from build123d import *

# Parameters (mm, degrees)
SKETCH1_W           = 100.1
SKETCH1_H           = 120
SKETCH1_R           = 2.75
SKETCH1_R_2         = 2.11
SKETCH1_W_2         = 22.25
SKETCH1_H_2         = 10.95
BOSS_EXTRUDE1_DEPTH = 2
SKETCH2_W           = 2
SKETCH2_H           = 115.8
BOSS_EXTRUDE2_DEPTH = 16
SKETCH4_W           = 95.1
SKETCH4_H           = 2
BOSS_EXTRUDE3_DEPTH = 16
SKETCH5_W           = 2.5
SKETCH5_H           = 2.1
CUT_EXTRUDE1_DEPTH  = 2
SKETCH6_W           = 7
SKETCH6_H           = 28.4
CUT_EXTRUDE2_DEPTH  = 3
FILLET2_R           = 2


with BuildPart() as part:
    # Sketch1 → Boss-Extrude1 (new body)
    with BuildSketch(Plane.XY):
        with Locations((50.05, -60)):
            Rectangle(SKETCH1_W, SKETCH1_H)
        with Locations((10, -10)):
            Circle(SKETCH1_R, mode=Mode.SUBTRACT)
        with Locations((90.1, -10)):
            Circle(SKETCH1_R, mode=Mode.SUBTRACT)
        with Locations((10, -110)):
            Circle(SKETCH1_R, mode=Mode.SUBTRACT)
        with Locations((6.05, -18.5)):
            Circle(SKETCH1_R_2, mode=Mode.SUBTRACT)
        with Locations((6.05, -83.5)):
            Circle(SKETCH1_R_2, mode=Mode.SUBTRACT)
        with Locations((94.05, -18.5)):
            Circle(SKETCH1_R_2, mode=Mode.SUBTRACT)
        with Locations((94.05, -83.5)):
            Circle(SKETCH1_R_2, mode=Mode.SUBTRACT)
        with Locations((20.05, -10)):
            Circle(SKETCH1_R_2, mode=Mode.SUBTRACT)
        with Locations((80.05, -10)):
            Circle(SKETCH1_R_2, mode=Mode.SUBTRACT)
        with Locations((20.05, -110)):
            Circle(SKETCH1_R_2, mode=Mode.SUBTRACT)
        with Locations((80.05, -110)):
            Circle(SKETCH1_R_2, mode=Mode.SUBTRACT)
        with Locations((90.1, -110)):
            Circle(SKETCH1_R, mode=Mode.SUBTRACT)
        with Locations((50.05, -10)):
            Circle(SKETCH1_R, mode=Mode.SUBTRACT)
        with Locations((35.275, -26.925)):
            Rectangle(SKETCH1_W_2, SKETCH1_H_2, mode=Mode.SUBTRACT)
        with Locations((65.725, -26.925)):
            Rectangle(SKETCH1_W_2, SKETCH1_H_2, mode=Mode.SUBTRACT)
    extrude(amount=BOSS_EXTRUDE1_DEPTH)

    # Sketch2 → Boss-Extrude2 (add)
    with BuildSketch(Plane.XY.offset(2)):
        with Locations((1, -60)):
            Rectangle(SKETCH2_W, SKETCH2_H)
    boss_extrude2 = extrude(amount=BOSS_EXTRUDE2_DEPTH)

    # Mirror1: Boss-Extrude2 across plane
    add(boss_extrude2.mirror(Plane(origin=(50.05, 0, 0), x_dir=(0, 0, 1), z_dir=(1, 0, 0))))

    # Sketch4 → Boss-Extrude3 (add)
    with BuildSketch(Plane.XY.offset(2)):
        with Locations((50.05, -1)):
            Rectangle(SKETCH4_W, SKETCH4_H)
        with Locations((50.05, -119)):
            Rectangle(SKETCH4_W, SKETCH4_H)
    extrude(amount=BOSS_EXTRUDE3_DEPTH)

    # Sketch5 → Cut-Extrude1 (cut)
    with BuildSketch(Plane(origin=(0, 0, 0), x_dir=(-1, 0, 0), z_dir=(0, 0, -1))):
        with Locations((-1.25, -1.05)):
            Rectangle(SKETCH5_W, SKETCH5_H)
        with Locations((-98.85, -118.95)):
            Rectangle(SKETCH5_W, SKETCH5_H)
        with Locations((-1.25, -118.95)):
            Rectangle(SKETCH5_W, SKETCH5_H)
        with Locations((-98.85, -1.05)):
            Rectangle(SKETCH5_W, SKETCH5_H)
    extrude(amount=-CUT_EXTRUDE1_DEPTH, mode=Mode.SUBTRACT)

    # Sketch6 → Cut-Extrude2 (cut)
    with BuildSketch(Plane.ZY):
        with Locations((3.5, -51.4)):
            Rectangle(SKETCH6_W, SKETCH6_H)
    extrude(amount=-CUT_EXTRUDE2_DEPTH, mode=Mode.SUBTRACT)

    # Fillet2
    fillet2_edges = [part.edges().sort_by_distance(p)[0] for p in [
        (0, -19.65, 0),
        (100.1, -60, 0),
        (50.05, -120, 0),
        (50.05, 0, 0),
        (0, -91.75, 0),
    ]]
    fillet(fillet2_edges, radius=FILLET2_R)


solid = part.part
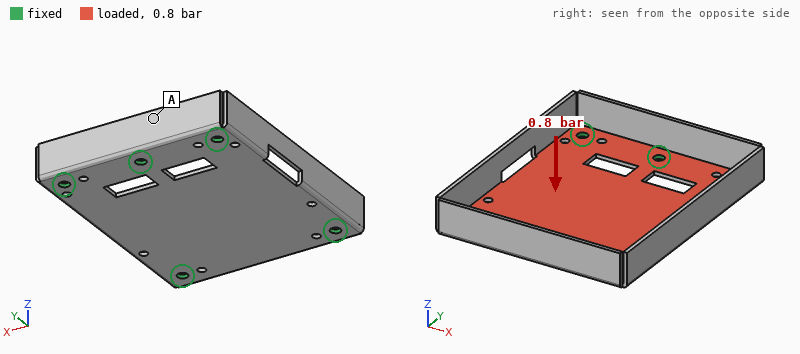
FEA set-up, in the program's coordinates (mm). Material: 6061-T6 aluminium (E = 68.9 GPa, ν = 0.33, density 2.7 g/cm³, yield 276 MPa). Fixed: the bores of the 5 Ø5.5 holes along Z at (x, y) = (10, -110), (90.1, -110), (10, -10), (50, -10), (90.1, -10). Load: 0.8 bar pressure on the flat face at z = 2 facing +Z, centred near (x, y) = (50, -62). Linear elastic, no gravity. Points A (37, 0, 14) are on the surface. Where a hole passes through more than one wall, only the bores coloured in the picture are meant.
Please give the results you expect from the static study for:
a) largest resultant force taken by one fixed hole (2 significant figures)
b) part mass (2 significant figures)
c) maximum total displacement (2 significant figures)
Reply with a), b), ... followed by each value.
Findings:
a) 230 N
b) 95 g
c) 0.40 mm
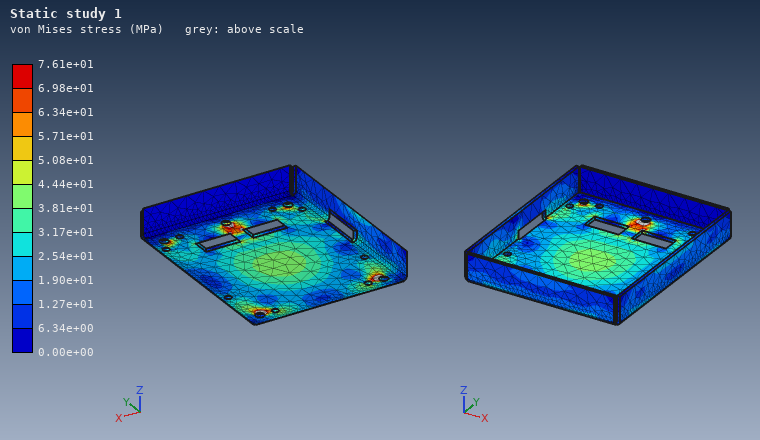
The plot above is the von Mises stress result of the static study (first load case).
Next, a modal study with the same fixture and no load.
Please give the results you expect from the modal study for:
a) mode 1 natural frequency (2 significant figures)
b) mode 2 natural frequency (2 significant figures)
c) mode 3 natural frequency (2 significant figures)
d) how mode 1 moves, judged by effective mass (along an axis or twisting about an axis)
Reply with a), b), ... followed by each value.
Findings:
a) 1200 Hz
b) 2300 Hz
c) 2500 Hz
d) along Z
